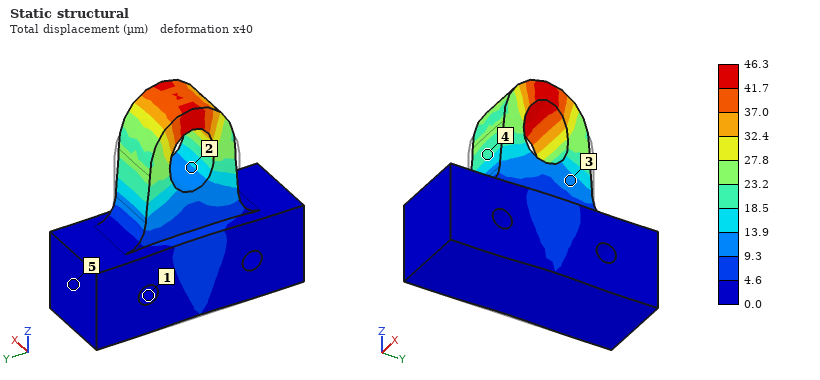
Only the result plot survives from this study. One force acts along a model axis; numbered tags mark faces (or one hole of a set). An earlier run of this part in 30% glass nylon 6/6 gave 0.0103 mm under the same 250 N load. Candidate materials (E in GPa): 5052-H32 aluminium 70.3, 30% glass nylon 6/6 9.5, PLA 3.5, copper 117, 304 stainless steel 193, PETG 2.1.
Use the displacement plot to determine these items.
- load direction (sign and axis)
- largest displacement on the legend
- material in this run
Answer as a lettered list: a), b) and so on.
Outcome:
a) +Z
b) 46.3 µm
c) PETG
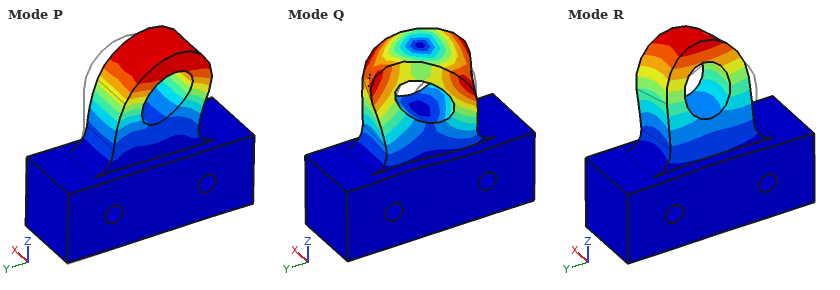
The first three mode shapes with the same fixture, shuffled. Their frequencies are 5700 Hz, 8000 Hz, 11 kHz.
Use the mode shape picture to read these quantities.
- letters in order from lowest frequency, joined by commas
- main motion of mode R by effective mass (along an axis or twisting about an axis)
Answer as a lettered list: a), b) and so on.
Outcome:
a) R, P, Q
b) along X
